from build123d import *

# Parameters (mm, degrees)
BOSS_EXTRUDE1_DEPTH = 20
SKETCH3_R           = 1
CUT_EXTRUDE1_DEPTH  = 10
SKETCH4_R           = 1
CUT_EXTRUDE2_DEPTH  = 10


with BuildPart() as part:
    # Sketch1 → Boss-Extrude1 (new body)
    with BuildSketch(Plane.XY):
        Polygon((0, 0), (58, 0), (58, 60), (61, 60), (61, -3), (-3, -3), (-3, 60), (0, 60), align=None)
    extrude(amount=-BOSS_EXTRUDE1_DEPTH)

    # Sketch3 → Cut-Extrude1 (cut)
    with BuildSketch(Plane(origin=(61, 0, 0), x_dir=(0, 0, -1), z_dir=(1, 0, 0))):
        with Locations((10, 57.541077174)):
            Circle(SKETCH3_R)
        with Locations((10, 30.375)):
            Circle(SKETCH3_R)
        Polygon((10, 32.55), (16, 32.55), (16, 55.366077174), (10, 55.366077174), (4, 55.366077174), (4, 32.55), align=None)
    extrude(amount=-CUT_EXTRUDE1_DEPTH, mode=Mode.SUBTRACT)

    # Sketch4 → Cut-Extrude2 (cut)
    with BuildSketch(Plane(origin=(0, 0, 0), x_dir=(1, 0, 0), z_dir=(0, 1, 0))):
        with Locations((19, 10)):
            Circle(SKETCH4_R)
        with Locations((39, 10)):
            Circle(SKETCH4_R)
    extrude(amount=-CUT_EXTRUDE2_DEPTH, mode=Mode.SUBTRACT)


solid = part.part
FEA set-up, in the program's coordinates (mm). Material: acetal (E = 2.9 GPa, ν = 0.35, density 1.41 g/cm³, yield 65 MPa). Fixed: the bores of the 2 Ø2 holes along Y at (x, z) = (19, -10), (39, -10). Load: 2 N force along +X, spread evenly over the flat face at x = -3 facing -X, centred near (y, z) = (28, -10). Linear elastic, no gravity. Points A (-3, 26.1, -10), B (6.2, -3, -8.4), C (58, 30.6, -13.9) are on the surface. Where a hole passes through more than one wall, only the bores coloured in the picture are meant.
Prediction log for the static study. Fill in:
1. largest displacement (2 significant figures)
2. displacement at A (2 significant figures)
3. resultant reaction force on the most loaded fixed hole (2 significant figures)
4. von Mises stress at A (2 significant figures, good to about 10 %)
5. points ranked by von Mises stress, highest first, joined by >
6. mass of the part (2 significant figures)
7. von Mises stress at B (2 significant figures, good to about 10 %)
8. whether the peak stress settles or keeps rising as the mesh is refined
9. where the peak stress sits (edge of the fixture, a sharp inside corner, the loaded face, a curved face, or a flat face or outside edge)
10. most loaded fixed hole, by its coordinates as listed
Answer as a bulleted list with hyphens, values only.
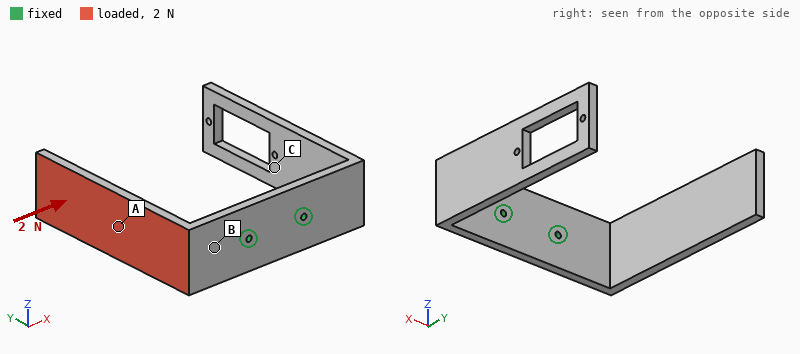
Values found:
- 0.98 mm
- 0.39 mm
- 2.0 N
- 0.61 MPa
- B > A > C
- 14 g
- 1.7 MPa
- keeps rising
- edge of the fixture
- (19, -10)
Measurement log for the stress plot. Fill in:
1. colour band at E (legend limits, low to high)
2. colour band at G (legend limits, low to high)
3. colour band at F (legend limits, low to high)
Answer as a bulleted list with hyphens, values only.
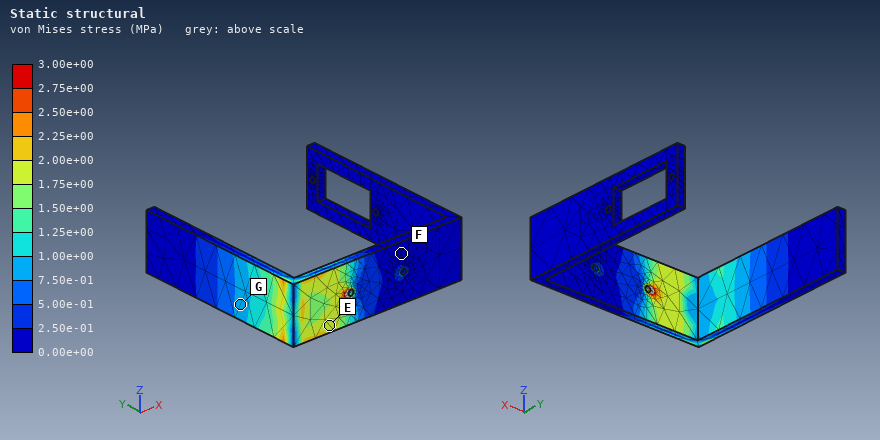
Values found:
- 1.75e+00 to 2.00e+00 MPa
- 7.50e-01 to 1.00e+00 MPa
- 0.00e+00 to 2.50e-01 MPa
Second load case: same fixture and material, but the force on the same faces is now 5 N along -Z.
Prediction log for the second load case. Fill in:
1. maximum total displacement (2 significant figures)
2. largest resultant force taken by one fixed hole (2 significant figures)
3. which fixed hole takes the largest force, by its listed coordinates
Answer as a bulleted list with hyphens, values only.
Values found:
- 1.0 mm
- 10.0 N
- (19, -10)
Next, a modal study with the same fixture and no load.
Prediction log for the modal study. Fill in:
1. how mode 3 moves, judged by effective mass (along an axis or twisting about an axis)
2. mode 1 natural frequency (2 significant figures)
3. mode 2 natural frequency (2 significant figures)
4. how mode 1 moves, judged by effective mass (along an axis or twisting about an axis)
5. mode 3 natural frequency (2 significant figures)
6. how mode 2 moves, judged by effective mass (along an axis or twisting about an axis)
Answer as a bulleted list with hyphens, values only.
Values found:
- along Z
- 120 Hz
- 150 Hz
- along X
- 180 Hz
- along X
